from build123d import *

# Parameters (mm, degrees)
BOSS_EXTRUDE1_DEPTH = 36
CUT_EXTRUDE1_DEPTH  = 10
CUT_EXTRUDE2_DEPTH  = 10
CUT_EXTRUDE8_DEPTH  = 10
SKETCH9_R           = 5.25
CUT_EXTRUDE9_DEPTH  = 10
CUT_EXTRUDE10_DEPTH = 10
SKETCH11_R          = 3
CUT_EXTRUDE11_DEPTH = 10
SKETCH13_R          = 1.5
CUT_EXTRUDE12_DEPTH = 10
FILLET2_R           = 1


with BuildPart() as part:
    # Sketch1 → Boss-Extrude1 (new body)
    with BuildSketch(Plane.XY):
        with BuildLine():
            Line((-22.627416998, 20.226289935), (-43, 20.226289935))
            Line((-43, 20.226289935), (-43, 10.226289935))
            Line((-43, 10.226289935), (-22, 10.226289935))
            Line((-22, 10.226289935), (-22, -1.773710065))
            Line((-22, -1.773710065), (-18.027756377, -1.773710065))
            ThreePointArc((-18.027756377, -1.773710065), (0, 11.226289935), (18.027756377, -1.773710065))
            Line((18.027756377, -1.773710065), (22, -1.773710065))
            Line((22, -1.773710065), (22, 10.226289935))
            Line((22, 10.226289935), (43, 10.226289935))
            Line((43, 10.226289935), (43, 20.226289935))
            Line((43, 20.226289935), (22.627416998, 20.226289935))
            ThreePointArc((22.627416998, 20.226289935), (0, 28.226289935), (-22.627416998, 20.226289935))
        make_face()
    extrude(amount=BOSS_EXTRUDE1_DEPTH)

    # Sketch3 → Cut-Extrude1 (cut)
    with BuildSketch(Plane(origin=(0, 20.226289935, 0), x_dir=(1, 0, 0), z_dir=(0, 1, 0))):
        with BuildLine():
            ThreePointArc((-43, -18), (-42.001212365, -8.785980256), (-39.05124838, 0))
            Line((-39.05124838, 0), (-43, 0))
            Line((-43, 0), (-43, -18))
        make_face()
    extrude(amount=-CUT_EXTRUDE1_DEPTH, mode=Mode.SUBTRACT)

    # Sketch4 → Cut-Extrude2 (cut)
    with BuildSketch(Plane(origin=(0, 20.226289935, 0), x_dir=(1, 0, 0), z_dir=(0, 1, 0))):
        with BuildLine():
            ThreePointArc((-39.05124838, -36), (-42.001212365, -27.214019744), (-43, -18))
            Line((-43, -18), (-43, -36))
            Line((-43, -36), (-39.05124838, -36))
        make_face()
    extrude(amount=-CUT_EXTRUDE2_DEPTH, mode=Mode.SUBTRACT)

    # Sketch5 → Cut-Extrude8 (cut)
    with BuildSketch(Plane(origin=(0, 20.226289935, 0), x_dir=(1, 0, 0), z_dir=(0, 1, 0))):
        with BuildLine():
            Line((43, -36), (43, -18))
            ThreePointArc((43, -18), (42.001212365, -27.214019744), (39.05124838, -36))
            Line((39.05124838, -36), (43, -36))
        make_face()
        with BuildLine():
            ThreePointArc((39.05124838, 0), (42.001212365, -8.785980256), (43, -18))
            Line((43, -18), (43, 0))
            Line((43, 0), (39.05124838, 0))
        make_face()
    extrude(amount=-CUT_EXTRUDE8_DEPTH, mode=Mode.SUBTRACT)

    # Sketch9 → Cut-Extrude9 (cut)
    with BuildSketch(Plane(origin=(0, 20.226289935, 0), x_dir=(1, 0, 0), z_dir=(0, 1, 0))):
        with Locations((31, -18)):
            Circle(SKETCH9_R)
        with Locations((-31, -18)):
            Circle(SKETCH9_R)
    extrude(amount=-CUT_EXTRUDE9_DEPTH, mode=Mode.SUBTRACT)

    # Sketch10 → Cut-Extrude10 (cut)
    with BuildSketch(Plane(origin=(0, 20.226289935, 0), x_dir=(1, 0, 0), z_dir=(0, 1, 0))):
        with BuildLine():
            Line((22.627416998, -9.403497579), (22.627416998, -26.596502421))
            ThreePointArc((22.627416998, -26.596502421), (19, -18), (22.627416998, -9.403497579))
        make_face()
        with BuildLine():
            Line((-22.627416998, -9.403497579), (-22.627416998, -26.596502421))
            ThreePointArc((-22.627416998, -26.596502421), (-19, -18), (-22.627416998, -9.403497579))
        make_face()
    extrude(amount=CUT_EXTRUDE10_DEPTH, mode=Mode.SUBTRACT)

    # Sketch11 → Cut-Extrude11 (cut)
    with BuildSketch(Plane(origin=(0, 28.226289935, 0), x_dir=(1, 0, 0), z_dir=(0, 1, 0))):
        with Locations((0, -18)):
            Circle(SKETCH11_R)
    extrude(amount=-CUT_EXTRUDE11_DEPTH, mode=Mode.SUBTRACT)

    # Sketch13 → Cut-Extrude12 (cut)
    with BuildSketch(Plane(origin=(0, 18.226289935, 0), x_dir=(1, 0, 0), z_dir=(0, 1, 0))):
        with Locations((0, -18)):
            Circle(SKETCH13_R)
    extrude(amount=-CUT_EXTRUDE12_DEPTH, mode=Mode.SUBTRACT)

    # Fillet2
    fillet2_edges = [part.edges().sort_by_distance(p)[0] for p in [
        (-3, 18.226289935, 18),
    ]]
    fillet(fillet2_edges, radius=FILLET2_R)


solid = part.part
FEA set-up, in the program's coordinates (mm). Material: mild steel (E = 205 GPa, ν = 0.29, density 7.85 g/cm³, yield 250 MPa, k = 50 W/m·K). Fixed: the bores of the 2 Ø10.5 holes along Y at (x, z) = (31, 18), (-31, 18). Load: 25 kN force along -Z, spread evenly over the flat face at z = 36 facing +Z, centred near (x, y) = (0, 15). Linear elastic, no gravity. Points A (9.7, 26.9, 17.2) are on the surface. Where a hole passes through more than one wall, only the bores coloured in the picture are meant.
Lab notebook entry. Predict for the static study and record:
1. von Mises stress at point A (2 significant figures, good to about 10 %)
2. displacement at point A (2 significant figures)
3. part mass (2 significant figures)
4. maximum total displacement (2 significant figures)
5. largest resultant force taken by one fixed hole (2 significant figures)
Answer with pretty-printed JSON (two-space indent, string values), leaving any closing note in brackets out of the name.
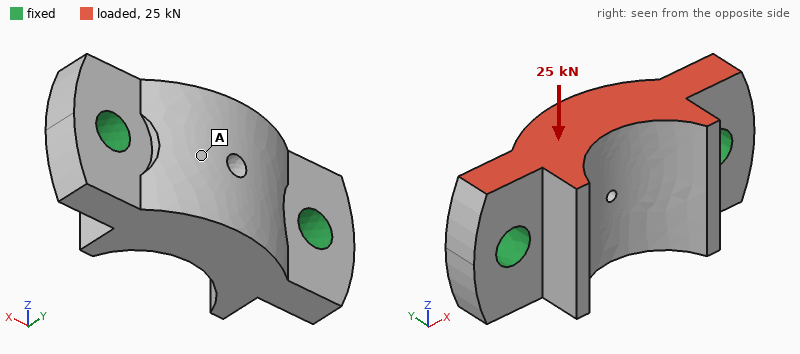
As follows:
{
  "von Mises stress at point A": "23 MPa",
  "displacement at point A": "8.8 µm",
  "part mass": "340 g",
  "maximum total displacement": "12 µm",
  "largest resultant force taken by one fixed hole": "13 kN"
}
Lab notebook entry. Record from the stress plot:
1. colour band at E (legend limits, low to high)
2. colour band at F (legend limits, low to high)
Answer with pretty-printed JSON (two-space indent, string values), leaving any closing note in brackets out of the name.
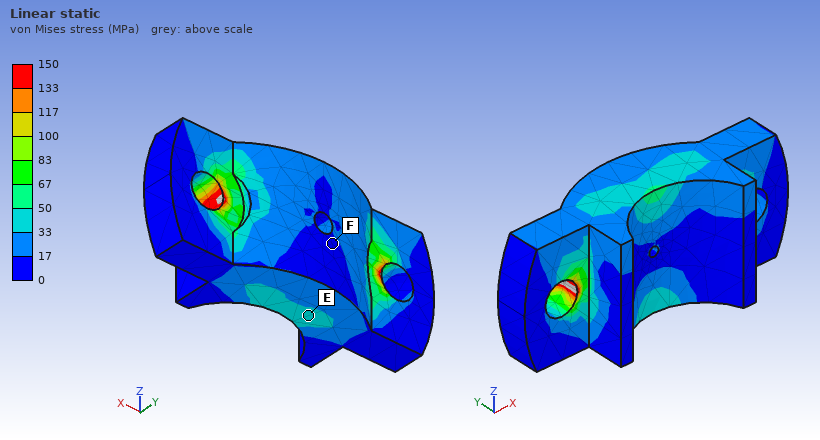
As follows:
{
  "colour band at E": "33 to 50 MPa",
  "colour band at F": "0 to 17 MPa"
}
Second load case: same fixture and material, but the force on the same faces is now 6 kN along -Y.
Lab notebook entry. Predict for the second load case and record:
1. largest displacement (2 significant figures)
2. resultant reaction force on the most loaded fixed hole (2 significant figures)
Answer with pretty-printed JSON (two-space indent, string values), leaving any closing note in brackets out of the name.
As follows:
{
  "largest displacement": "16 µm",
  "resultant reaction force on the most loaded fixed hole": "3.1 kN"
}
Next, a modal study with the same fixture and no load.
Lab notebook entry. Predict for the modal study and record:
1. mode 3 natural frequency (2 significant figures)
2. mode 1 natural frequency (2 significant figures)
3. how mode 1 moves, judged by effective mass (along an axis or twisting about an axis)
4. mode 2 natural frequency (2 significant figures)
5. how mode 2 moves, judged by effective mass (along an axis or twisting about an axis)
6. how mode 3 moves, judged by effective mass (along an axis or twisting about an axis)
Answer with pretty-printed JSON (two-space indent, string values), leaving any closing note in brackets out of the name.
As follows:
{
  "mode 3 natural frequency": "16 kHz",
  "mode 1 natural frequency": "11 kHz",
  "how mode 1 moves, judged by effective mass": "twisting about X",
  "mode 2 natural frequency": "12 kHz",
  "how mode 2 moves, judged by effective mass": "along Y",
  "how mode 3 moves, judged by effective mass": "along Z"
}
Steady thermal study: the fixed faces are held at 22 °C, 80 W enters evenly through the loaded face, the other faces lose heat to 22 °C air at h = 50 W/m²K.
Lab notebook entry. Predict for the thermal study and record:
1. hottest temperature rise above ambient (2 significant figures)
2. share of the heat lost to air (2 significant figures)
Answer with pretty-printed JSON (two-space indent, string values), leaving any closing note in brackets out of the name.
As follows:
{
  "hottest temperature rise above ambient": "42 K",
  "share of the heat lost to air": "9.4 %"
}
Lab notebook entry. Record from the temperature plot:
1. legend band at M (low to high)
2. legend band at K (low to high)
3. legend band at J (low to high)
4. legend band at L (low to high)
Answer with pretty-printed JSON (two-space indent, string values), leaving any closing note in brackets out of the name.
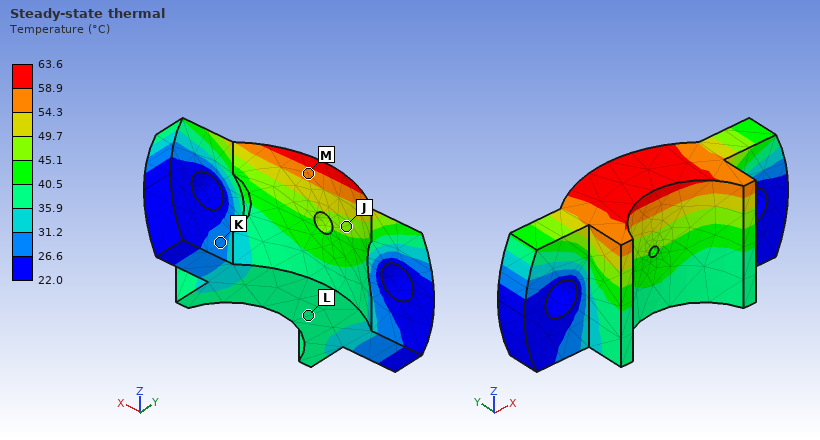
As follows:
{
  "legend band at M": "54.3 to 58.9 °C",
  "legend band at K": "26.6 to 31.2 °C",
  "legend band at J": "45.1 to 49.7 °C",
  "legend band at L": "35.9 to 40.5 °C"
}
